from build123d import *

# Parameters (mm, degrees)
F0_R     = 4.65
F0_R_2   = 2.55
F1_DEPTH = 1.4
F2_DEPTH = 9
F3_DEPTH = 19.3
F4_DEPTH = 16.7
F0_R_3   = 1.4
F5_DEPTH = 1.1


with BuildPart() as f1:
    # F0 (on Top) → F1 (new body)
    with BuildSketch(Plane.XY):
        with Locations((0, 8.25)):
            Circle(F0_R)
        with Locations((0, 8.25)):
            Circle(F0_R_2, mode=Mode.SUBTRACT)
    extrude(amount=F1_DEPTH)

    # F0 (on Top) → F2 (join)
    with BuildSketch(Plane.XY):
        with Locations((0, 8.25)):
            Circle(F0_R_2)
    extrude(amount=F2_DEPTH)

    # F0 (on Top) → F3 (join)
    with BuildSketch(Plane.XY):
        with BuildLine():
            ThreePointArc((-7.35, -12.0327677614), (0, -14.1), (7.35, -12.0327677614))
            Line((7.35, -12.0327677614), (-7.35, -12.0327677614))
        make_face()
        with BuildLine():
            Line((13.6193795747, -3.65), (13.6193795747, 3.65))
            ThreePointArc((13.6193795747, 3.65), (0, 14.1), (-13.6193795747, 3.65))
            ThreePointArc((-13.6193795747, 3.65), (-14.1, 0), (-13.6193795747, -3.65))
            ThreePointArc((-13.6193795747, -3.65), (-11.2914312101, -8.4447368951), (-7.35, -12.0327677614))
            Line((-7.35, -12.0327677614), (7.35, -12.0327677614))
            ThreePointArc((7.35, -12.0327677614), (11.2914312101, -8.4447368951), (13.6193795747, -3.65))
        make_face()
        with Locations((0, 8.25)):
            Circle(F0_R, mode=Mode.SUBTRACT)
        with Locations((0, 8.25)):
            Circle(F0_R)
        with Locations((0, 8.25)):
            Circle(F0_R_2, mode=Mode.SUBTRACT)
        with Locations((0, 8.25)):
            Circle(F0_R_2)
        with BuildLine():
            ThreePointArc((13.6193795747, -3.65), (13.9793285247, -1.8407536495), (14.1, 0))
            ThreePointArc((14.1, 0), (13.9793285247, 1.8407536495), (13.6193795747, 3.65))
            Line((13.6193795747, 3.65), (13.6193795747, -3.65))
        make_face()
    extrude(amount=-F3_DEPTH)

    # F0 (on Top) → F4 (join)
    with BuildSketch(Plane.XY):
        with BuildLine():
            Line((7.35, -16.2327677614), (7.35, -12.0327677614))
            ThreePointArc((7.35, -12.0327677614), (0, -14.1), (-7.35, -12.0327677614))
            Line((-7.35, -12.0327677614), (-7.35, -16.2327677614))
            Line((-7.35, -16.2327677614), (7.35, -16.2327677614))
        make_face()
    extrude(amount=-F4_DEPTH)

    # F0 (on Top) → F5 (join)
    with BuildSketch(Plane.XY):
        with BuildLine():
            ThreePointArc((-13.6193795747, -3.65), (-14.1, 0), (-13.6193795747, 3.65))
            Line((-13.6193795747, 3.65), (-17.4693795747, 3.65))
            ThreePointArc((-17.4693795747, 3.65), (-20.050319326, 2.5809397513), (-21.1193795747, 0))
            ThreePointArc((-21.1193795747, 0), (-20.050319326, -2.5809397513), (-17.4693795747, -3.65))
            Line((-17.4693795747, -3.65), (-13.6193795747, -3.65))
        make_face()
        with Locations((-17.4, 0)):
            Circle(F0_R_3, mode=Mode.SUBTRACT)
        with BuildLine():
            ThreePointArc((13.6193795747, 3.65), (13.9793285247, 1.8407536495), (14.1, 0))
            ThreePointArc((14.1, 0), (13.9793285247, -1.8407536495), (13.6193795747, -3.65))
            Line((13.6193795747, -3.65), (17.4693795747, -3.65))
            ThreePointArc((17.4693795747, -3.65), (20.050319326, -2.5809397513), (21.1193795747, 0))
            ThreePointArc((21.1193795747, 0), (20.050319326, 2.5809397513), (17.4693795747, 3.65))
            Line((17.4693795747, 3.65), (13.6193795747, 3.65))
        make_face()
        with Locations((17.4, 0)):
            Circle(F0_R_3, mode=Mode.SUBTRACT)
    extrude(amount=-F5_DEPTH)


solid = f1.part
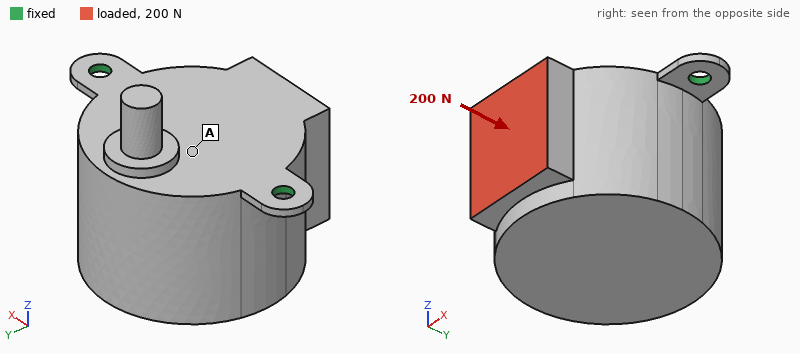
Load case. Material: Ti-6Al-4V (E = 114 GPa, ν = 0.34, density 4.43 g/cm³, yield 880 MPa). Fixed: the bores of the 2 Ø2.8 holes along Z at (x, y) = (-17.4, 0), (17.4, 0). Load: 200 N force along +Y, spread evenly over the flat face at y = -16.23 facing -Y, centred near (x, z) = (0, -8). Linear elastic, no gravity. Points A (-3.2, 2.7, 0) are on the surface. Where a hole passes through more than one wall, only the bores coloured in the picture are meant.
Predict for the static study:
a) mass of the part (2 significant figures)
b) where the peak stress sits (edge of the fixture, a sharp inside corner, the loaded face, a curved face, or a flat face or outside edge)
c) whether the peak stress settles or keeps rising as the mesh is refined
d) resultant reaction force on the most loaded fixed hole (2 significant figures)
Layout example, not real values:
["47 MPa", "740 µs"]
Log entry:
["58 g", "edge of the fixture", "keeps rising", "100 N"]
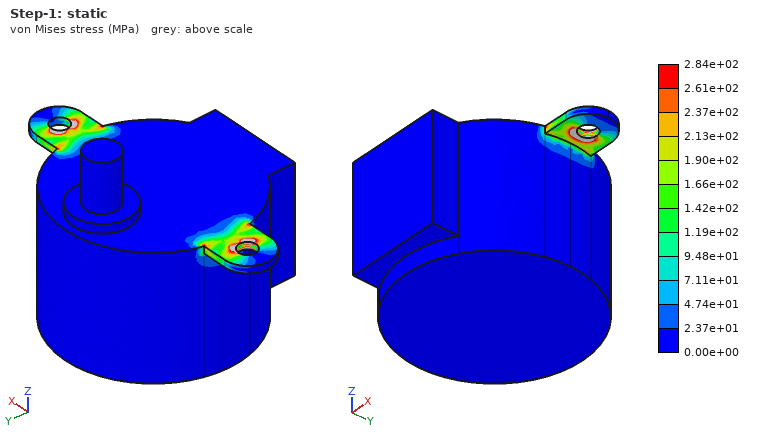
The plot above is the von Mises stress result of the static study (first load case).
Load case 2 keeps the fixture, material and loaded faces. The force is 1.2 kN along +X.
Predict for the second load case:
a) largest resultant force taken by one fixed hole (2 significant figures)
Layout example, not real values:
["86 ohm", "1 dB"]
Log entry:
["910 N"]
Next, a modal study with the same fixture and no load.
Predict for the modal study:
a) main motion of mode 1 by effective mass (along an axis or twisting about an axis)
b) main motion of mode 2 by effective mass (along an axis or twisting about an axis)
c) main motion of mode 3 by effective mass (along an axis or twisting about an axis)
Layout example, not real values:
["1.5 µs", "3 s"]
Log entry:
["along Y", "along Z", "along X"]
